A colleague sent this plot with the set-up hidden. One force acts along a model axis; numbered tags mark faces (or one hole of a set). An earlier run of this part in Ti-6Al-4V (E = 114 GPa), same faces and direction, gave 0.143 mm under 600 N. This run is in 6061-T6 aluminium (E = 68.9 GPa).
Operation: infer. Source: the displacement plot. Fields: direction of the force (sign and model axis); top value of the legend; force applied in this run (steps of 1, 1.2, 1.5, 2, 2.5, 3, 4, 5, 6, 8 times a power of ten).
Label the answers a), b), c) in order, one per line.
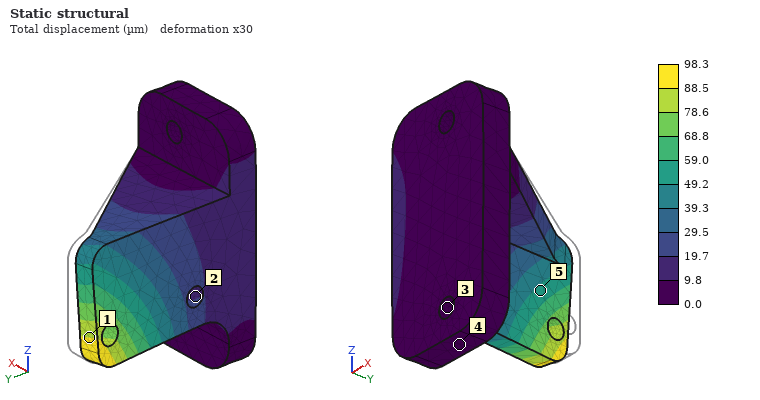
a) -X
b) 98.3 µm
c) 250 N
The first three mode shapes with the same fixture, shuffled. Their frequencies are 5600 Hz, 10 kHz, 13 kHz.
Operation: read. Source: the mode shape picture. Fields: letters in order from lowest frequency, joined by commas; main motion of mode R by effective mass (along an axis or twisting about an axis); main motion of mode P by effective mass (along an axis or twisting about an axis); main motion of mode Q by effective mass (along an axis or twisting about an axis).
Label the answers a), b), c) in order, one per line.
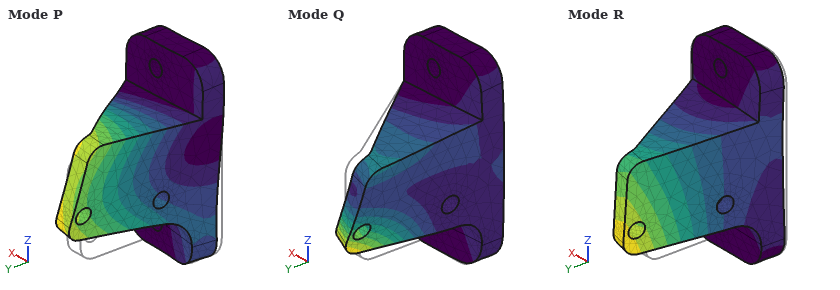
a) R, P, Q
b) along X
c) along Z
d) along Y
